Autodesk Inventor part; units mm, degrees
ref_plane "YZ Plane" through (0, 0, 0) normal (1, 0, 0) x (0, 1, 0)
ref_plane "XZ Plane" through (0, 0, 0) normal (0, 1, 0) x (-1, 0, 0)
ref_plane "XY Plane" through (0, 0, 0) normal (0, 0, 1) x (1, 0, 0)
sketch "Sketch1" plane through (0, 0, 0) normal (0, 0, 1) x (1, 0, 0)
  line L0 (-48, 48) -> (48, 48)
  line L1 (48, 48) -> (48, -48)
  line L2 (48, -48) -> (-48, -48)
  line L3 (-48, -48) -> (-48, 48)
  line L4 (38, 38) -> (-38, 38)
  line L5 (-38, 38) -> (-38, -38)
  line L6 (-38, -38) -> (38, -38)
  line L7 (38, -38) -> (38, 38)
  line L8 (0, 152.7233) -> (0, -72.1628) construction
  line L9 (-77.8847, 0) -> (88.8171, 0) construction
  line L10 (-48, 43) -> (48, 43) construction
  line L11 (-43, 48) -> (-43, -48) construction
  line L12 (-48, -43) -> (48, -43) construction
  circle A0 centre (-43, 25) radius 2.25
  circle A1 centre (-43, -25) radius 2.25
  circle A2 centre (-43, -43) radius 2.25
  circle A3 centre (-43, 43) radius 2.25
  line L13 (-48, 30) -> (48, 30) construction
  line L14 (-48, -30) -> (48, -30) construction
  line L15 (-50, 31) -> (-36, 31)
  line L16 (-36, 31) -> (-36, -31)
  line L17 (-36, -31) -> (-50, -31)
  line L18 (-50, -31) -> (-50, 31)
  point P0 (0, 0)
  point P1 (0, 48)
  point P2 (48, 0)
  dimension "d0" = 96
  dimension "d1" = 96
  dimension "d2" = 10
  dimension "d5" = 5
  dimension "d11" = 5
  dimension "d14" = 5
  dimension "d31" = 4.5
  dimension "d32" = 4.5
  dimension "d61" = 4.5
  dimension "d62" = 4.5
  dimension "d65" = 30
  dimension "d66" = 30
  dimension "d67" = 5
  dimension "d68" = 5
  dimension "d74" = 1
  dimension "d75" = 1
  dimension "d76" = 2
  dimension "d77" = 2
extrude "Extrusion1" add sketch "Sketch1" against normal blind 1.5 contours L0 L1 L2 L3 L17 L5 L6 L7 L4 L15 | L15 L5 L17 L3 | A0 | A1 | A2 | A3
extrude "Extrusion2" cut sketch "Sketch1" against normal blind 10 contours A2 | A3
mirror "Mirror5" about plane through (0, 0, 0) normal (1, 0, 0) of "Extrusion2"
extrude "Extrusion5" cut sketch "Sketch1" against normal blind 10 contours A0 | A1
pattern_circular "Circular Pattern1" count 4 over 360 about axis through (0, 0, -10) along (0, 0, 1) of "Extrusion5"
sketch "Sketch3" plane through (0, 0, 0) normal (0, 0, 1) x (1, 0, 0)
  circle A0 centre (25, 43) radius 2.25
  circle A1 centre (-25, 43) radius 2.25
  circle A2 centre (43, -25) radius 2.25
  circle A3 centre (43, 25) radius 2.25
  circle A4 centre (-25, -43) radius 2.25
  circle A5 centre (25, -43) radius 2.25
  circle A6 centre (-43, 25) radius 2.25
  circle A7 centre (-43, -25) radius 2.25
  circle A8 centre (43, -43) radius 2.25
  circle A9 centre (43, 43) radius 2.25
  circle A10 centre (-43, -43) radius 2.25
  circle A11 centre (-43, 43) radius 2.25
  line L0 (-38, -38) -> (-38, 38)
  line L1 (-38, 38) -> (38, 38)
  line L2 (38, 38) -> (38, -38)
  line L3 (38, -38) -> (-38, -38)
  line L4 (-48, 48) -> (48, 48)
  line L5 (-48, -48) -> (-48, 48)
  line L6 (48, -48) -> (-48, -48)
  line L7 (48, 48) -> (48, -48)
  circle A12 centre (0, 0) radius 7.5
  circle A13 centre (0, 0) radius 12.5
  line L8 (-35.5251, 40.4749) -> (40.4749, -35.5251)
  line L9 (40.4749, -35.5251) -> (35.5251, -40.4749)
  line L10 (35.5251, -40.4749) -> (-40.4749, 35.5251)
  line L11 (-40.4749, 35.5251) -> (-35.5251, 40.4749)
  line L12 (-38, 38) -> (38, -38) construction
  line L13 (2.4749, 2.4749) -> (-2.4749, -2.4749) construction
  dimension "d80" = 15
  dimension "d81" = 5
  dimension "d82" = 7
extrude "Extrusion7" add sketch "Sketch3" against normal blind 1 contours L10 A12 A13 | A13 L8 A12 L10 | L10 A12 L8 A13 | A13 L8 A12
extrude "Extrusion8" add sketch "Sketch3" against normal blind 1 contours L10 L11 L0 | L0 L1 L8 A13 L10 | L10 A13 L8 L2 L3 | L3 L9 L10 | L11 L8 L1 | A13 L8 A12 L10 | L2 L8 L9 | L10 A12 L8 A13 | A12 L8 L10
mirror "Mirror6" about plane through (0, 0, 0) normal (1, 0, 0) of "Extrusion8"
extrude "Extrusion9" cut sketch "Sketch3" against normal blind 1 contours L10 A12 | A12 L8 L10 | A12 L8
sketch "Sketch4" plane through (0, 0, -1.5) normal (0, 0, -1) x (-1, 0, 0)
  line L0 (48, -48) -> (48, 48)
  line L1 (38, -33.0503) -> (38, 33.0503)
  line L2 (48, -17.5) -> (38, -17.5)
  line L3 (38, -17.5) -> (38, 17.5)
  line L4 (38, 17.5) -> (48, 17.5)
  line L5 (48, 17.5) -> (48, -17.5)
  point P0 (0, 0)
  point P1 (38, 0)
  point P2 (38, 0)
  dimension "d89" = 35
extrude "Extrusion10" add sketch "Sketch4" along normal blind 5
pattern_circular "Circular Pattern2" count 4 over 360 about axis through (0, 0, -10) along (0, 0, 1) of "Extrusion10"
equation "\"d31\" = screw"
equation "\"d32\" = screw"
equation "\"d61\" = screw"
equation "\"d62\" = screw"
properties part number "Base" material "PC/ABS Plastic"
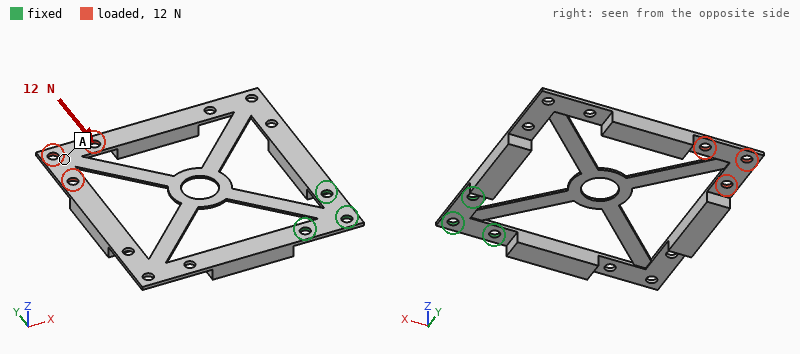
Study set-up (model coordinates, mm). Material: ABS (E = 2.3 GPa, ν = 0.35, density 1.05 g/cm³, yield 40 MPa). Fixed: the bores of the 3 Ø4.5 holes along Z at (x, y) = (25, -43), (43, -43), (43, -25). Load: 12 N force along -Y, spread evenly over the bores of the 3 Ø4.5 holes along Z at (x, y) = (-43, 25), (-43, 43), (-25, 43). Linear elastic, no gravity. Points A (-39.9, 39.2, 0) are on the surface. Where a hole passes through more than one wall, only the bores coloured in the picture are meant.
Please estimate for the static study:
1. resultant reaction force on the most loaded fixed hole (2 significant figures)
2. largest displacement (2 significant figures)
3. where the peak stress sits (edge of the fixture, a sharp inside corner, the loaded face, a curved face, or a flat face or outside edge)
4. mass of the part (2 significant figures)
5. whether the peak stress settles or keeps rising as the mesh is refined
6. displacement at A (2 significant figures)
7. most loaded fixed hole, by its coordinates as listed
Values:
16 N
1.5 mm
edge of the fixture
14 g
keeps rising
1.3 mm
(25, -43)
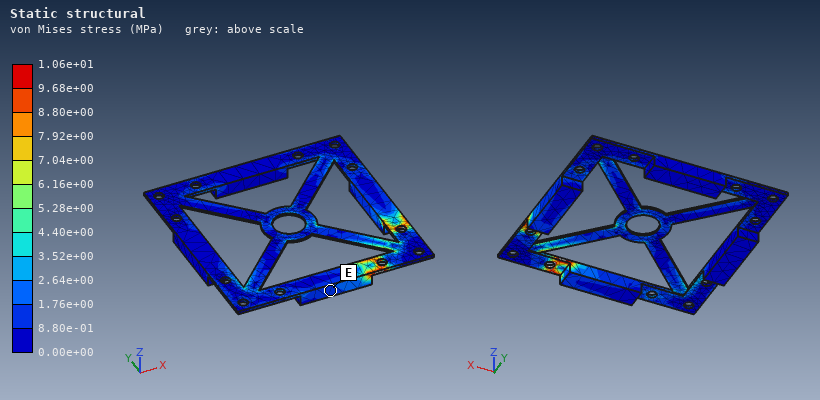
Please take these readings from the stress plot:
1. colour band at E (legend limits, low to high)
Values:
8.80e-01 to 1.76e+00 MPa
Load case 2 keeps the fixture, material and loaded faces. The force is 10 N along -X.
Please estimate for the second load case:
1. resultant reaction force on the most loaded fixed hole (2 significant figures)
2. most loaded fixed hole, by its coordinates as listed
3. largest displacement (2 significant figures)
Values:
14 N
(43, -25)
1.2 mm
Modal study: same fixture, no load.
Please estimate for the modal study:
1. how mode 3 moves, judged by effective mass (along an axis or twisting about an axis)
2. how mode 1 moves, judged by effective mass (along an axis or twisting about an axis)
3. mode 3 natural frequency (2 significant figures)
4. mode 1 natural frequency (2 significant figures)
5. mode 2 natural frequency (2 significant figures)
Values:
along Z
along Z
100 Hz
24 Hz
59 Hz
